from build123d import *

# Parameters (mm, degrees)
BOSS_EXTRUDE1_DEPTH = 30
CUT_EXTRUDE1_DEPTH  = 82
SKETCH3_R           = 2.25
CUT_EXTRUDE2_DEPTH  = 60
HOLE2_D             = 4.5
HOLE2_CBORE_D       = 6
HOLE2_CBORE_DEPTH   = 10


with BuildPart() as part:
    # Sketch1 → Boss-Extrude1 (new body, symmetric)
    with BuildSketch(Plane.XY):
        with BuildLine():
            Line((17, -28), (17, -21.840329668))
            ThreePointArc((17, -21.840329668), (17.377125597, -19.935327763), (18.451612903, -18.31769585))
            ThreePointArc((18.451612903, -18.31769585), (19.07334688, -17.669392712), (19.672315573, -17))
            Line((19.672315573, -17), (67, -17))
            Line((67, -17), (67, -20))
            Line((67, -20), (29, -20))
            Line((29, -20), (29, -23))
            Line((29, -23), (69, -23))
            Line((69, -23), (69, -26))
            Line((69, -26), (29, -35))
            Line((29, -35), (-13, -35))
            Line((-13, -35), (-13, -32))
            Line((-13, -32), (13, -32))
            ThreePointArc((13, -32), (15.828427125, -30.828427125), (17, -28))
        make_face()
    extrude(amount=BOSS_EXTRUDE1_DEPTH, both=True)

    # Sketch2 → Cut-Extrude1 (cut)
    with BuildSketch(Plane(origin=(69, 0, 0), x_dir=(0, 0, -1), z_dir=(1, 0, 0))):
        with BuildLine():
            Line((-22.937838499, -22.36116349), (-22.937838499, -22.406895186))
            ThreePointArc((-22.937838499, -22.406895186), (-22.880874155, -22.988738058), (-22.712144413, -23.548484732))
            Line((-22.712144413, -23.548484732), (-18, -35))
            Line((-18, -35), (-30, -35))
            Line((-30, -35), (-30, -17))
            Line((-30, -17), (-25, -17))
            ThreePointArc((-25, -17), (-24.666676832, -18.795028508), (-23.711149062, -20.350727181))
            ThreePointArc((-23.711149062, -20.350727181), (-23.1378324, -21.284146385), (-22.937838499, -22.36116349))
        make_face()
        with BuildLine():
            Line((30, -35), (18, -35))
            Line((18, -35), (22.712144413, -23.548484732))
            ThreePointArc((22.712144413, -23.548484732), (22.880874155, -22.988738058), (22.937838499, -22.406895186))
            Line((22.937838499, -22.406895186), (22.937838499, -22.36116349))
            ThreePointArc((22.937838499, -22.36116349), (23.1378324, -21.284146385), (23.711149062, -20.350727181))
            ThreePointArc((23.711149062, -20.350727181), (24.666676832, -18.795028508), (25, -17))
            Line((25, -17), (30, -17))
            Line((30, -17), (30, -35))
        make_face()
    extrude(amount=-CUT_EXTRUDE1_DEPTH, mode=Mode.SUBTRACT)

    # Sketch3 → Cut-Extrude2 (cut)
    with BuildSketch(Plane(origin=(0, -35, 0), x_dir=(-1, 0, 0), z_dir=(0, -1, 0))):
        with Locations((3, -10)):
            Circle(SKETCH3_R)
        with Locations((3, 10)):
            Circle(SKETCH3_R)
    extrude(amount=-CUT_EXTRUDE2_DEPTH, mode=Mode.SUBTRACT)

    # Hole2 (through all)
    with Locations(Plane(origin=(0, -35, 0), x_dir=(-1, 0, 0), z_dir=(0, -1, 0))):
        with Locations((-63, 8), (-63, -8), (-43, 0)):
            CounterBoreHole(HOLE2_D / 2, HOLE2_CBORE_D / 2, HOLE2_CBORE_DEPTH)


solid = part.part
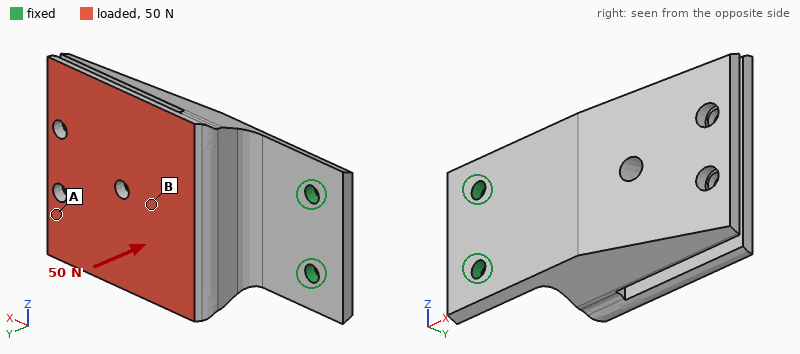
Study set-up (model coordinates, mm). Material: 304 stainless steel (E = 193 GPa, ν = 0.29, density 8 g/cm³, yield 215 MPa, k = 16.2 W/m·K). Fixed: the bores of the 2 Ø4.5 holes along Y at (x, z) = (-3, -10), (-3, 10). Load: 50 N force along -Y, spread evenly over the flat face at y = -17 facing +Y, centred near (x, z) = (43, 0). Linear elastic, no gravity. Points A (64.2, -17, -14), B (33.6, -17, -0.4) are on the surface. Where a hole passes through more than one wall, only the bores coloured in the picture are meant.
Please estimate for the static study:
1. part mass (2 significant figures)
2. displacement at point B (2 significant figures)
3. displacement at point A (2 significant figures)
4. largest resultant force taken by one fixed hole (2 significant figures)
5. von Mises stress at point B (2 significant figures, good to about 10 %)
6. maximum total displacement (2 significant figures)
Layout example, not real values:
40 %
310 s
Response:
240 g
0.064 mm
0.13 mm
25 N
7.2 MPa
0.14 mm
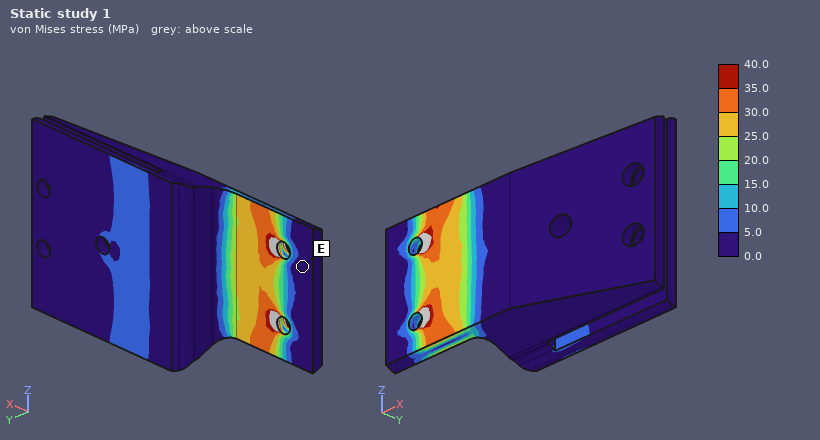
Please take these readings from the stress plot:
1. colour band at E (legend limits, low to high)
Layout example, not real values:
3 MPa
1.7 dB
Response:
0.0 to 5.0 MPa
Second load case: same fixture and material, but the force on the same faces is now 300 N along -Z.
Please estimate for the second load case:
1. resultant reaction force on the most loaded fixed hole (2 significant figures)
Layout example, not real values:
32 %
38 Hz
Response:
650 N
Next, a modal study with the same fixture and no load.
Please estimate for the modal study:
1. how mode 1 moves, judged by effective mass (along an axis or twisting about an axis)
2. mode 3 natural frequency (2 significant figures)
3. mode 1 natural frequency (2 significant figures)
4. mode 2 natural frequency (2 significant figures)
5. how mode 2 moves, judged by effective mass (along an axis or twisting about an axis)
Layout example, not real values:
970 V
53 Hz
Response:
along Y
1800 Hz
290 Hz
1300 Hz
along Z
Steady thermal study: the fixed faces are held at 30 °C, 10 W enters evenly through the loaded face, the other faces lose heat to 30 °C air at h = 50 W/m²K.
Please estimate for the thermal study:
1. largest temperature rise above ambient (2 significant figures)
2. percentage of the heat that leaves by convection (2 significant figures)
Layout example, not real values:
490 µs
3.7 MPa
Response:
46 K
90 %
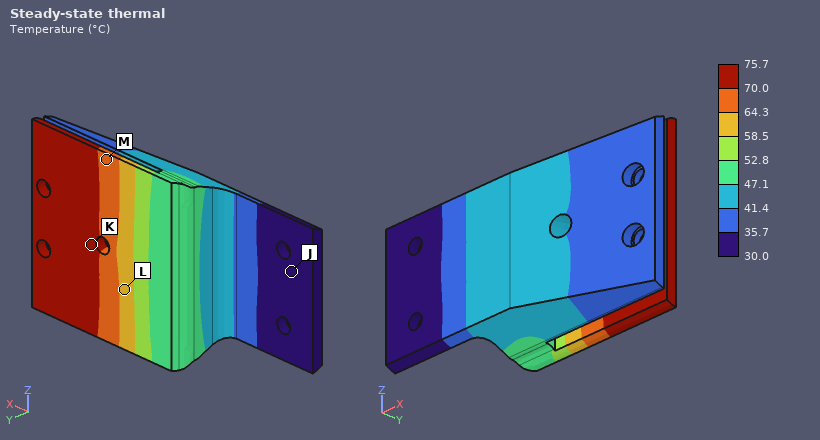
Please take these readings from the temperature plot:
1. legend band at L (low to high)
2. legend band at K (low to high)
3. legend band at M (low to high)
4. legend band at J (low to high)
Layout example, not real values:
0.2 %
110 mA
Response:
58.5 to 64.3 °C
70.0 to 75.7 °C
64.3 to 70.0 °C
30.0 to 35.7 °C
